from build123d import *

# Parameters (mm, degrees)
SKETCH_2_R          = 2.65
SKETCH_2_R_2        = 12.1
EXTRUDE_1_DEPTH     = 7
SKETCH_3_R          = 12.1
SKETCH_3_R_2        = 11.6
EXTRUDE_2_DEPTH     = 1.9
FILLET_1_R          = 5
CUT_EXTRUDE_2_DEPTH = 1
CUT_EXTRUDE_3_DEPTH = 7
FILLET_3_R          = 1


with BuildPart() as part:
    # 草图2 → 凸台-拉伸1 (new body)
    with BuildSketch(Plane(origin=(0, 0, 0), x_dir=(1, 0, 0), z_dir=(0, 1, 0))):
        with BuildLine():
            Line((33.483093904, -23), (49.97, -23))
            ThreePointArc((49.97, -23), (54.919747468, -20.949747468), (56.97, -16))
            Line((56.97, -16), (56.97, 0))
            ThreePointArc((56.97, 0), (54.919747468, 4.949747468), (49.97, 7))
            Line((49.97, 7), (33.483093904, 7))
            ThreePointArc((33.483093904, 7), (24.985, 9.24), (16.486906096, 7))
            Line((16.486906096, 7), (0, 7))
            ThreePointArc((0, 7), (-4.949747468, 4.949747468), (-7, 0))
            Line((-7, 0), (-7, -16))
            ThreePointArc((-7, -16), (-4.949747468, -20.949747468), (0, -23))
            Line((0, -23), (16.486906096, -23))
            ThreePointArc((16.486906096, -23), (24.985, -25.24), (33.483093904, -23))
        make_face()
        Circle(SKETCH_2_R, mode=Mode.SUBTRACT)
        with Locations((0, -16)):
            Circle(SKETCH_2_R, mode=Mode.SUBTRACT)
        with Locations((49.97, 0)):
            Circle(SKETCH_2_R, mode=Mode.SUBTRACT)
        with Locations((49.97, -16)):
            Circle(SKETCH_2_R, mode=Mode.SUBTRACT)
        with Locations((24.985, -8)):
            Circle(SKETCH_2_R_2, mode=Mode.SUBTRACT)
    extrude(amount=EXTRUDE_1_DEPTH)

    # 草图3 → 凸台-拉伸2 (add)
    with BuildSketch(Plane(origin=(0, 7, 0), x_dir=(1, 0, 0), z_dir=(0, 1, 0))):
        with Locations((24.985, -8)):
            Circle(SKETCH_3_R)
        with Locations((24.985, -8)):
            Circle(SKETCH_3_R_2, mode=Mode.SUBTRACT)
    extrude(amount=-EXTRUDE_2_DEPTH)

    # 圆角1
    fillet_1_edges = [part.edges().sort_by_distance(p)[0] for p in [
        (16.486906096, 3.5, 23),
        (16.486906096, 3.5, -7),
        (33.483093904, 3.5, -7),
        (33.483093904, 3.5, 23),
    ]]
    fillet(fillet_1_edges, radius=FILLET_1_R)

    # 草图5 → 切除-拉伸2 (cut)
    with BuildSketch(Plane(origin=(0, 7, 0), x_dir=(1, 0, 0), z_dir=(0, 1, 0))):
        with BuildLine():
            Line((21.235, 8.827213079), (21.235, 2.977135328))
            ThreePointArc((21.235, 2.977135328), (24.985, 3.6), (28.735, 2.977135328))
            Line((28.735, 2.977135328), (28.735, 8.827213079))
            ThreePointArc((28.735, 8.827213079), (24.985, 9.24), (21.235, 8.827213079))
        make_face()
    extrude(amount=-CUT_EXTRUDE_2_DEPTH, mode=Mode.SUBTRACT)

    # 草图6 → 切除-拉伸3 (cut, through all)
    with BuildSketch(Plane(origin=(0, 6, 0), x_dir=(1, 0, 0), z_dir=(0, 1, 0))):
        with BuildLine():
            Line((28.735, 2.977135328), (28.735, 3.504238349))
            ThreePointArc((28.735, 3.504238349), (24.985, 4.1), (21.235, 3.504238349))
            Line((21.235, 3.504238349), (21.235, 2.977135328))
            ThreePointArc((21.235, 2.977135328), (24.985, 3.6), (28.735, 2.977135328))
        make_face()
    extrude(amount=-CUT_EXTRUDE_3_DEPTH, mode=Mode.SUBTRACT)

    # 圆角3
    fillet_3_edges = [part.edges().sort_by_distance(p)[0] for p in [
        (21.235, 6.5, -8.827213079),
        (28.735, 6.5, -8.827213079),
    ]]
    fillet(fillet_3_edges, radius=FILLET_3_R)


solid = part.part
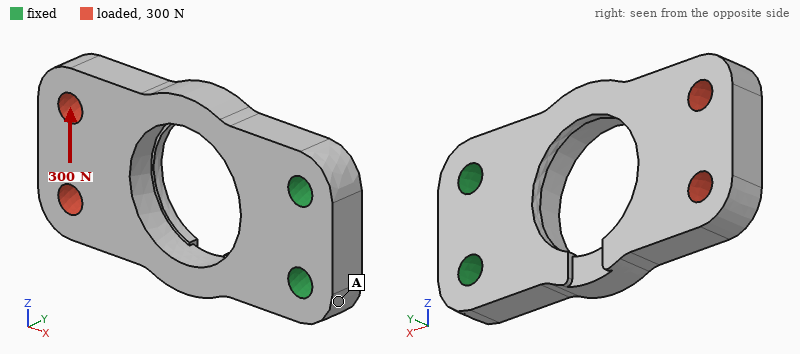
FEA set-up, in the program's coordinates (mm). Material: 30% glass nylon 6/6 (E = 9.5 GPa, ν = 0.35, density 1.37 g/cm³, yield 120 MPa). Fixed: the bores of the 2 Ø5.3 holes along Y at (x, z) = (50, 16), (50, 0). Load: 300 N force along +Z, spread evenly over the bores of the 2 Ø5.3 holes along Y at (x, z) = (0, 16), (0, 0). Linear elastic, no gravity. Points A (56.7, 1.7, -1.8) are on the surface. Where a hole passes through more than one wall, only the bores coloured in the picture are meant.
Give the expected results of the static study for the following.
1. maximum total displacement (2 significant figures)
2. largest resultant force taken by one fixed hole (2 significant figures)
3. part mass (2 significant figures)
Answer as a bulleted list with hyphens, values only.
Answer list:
- 0.37 mm
- 750 N
- 13 g
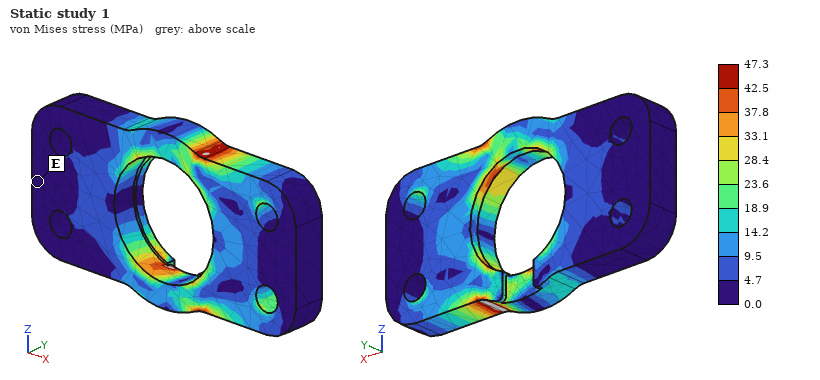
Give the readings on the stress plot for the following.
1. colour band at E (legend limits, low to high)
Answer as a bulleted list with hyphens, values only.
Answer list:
- 0.0 to 4.7 MPa
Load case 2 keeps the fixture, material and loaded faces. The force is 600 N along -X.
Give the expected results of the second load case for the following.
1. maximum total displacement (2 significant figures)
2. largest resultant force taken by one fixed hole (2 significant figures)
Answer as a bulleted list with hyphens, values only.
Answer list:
- 59 µm
- 310 N
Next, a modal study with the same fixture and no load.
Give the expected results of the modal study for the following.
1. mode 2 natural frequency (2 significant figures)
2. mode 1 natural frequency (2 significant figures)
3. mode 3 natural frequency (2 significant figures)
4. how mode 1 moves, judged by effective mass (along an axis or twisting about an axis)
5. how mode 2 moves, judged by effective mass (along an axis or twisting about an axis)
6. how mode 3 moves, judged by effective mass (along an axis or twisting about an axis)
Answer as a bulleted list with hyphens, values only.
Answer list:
- 2000 Hz
- 750 Hz
- 2700 Hz
- along Y
- along Z
- twisting about X
